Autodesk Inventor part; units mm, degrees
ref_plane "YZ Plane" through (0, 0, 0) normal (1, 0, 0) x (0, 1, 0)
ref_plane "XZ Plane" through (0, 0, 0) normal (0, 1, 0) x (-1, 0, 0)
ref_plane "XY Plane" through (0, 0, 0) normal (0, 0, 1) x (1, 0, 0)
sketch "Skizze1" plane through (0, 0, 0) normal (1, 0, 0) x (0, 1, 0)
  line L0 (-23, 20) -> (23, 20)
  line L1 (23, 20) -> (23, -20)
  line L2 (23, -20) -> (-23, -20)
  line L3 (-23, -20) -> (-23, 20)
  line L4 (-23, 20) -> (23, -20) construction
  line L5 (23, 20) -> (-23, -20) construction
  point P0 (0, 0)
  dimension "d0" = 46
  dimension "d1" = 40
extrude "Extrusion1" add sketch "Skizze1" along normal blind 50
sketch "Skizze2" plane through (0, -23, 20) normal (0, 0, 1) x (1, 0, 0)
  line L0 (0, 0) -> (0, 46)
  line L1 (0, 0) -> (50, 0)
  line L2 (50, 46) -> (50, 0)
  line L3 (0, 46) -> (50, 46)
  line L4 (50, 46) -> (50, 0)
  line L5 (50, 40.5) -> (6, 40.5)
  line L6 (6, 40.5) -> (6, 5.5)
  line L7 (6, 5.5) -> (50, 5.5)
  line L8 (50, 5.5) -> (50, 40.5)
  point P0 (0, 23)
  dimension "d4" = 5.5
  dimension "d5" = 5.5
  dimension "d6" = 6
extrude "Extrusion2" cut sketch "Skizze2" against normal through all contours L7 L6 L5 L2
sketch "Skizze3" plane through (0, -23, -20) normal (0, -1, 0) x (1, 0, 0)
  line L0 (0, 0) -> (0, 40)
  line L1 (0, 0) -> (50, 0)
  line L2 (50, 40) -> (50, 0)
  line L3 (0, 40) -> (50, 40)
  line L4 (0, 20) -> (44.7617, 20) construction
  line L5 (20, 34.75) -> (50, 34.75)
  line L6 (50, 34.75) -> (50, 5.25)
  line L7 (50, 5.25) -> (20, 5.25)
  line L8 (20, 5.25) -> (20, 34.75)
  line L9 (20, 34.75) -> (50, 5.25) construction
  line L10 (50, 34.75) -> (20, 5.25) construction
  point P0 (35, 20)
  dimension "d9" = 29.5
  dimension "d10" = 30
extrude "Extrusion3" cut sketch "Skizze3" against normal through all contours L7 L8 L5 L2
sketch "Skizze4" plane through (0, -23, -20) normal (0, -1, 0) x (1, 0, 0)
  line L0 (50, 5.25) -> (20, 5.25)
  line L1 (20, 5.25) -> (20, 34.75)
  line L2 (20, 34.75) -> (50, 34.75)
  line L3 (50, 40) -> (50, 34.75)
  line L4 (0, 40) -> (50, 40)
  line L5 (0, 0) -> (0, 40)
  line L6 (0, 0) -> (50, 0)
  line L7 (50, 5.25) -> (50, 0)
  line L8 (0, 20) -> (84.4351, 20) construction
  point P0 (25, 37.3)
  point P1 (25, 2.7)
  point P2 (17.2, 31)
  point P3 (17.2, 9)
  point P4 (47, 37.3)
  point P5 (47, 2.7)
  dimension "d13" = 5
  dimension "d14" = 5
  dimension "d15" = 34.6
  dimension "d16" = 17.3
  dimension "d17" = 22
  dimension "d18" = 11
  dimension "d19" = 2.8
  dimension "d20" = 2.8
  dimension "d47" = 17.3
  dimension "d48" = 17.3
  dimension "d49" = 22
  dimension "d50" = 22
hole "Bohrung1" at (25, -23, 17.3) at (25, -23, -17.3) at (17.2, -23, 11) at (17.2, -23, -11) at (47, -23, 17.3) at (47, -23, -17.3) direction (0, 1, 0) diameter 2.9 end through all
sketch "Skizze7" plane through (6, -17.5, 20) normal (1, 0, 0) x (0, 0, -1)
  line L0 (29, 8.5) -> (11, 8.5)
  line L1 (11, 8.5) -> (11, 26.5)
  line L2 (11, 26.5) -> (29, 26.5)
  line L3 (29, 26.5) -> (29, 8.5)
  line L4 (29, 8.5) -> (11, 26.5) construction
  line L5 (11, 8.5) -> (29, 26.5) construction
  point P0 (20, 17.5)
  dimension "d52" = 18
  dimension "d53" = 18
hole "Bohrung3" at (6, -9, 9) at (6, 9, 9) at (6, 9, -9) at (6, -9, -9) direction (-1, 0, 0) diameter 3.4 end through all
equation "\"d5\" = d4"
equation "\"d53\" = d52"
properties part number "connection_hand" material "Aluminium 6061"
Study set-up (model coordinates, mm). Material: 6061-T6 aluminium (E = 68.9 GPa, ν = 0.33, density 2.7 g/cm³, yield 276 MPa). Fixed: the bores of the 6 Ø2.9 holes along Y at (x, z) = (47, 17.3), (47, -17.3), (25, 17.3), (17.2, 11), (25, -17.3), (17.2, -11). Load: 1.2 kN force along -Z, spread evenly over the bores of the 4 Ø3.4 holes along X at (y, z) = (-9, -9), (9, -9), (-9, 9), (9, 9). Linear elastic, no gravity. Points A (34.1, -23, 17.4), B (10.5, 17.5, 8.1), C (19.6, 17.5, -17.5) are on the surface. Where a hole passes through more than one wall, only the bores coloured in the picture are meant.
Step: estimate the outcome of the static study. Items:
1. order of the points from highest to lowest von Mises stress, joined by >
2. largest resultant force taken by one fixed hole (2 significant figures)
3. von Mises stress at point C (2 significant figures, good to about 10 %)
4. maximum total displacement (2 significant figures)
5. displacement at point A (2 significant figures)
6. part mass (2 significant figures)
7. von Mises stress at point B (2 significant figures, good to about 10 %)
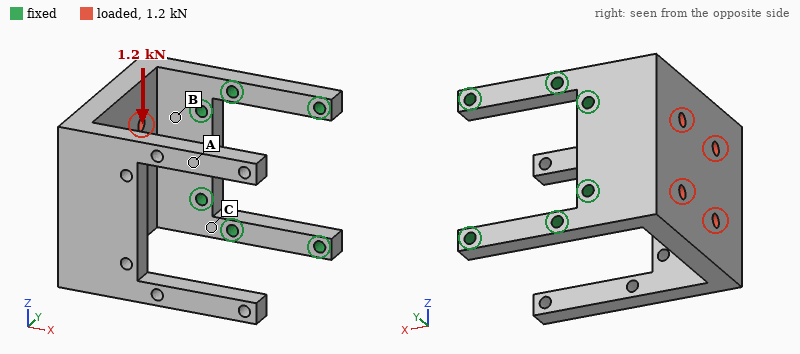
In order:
B > C > A
1.2 kN
32 MPa
0.17 mm
0.15 mm
54 g
51 MPa
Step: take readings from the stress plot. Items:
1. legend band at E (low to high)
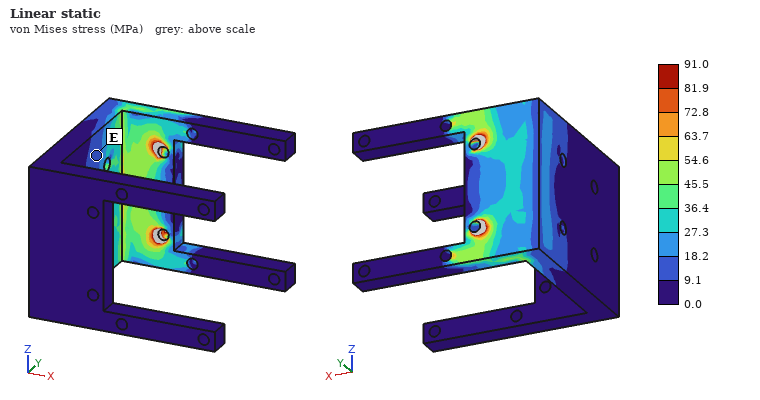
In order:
9.1 to 18.2 MPa
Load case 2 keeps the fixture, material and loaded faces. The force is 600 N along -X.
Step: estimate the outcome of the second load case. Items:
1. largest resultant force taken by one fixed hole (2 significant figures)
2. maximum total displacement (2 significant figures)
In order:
330 N
0.42 mm
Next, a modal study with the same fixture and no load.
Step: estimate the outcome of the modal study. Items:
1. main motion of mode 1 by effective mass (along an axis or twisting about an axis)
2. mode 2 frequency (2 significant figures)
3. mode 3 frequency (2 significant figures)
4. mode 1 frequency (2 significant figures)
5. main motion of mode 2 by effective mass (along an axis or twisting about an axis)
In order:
along X
1700 Hz
2500 Hz
960 Hz
along Z
